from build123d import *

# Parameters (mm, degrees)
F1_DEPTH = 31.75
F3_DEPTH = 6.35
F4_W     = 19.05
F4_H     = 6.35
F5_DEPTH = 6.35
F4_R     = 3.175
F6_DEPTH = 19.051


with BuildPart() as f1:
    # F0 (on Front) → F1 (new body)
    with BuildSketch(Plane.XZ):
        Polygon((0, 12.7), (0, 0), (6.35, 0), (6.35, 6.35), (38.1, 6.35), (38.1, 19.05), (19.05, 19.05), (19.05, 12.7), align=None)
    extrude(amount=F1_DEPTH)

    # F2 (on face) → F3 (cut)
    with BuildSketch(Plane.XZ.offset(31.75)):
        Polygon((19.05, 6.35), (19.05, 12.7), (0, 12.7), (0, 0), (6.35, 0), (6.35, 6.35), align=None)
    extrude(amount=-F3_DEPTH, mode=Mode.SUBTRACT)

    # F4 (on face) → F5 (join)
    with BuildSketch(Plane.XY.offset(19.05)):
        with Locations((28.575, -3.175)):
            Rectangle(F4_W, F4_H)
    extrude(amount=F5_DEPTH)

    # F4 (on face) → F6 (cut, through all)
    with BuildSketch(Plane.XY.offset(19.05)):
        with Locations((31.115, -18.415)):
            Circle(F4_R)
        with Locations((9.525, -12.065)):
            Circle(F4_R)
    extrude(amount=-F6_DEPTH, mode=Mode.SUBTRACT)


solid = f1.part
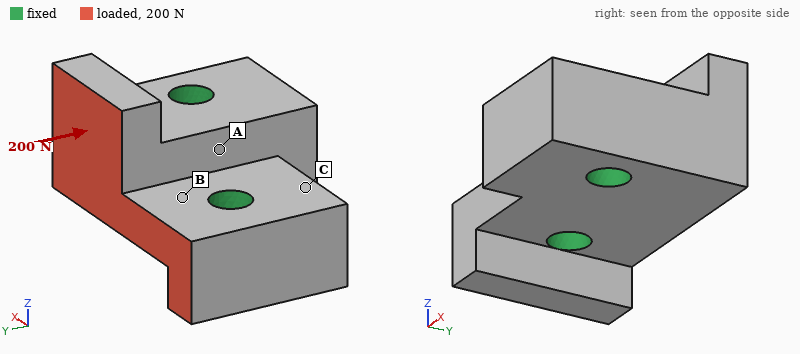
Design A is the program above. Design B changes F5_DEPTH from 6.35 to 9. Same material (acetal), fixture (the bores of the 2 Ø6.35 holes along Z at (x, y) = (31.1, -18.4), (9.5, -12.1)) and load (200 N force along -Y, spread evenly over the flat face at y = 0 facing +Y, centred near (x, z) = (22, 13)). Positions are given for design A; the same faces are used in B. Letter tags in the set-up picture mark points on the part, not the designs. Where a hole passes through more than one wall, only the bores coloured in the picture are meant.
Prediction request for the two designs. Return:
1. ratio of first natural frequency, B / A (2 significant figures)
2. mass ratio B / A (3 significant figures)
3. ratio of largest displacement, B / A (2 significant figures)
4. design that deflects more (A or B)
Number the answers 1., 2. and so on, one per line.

1. 0.87
2. 1.03
3. 1.8
4. B
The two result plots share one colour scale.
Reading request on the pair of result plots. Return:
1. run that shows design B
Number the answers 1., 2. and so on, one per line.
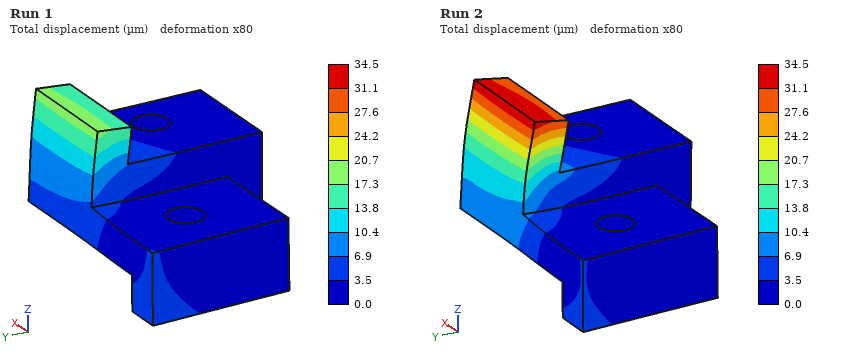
1. Run 2
